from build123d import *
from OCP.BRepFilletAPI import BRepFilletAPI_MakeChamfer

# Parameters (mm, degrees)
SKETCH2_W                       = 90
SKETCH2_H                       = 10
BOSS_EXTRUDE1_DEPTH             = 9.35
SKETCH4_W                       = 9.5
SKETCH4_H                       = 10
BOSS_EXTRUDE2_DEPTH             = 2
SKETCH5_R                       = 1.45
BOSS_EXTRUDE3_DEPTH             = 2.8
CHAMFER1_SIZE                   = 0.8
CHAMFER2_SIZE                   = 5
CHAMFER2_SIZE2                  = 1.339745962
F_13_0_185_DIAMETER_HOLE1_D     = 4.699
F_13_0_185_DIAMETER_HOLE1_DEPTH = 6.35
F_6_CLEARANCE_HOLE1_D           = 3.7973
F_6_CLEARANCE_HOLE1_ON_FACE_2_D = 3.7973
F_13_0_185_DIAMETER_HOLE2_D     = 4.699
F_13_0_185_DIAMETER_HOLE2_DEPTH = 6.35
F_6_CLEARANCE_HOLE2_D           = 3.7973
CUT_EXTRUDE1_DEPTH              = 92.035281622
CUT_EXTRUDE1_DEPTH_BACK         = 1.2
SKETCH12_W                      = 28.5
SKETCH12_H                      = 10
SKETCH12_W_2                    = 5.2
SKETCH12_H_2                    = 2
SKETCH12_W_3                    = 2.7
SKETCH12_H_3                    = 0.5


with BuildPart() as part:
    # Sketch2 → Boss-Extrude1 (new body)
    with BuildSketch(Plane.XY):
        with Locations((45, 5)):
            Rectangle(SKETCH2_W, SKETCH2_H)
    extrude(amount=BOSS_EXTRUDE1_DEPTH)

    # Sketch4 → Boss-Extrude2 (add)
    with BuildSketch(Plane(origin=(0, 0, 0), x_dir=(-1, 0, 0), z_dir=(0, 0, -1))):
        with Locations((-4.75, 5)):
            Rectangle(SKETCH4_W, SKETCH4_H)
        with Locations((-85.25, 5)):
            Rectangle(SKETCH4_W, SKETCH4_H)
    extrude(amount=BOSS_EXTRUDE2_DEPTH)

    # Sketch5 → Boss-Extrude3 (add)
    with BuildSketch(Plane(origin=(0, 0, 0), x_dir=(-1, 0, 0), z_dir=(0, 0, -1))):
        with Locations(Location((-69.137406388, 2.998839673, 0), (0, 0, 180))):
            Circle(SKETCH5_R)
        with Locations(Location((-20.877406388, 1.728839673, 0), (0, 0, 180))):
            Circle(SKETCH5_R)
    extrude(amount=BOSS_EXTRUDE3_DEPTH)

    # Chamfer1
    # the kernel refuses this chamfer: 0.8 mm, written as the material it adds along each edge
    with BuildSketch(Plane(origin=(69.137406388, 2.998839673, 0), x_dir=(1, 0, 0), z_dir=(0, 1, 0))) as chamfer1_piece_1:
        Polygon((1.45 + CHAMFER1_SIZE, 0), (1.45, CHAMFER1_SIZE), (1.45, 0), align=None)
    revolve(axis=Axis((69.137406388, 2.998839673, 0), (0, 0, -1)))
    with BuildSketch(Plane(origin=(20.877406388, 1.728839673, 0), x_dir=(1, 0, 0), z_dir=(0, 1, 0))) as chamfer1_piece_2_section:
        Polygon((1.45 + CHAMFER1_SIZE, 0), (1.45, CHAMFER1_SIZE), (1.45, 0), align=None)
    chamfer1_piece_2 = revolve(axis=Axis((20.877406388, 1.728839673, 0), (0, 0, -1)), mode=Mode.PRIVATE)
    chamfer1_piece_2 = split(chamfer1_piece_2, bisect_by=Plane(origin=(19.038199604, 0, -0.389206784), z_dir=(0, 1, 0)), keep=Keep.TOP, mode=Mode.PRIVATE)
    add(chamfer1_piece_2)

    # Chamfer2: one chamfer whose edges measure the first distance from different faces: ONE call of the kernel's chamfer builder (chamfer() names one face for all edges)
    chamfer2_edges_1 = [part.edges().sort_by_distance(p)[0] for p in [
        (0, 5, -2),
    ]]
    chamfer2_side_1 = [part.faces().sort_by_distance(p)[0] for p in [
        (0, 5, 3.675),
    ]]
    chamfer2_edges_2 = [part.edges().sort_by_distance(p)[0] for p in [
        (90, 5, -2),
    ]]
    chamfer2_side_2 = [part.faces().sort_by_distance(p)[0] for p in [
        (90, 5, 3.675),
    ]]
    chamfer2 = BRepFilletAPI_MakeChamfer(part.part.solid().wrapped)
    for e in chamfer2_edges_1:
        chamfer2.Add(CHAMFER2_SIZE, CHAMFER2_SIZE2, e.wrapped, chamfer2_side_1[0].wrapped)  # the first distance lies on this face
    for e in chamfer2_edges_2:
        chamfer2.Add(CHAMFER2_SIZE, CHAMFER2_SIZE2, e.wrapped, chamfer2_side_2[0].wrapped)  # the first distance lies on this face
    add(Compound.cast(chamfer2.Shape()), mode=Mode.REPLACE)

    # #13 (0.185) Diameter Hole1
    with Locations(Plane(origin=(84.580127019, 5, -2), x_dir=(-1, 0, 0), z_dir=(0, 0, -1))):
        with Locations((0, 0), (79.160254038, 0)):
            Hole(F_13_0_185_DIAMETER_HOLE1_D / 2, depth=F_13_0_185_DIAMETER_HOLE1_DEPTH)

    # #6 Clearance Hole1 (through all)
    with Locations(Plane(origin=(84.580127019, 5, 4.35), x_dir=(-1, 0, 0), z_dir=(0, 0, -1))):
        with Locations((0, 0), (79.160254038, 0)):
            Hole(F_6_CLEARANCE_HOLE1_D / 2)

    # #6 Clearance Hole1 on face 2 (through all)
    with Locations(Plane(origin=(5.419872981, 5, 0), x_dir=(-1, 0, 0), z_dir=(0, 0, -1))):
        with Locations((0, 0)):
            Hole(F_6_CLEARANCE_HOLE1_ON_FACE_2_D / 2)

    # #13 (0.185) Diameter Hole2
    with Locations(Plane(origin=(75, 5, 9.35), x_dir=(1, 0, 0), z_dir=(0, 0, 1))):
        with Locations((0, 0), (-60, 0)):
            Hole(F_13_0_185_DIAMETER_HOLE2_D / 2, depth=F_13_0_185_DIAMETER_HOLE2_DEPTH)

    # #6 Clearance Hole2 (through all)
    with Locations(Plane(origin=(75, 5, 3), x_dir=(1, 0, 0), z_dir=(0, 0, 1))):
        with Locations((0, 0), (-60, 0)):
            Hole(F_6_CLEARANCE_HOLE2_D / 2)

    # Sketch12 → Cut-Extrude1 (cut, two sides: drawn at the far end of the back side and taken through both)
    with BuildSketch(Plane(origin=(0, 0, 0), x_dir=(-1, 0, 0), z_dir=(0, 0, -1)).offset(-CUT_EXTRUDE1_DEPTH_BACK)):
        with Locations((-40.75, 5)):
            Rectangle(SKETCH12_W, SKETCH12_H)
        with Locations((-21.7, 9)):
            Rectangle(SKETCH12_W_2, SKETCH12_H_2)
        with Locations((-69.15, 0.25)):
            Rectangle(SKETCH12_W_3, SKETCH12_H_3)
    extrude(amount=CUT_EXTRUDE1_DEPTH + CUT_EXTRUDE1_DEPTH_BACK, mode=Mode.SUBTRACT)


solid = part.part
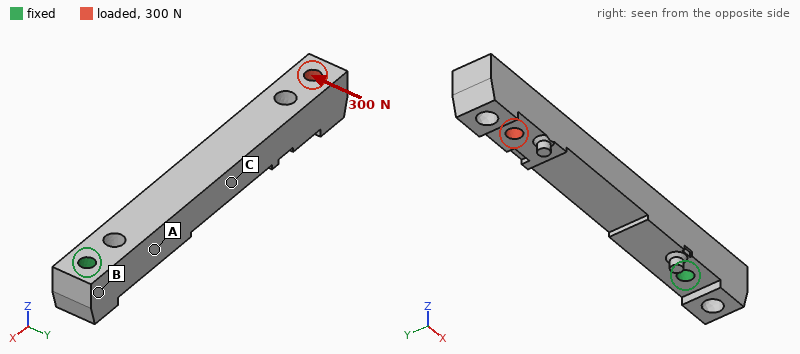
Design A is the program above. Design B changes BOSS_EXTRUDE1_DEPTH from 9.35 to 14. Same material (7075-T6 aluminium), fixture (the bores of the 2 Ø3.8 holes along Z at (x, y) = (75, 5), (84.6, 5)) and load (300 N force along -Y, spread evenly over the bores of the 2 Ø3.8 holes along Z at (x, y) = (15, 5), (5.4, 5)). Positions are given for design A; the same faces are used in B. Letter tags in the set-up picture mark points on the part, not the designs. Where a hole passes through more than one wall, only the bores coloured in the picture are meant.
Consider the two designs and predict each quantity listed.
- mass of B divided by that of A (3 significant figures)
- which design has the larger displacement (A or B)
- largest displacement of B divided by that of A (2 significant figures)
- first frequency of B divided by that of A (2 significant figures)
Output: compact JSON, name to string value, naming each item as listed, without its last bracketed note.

{"mass of B divided by that of A": "1.50", "which design has the larger displacement": "A", "largest displacement of B divided by that of A": "0.72", "first frequency of B divided by that of A": "1.1"}
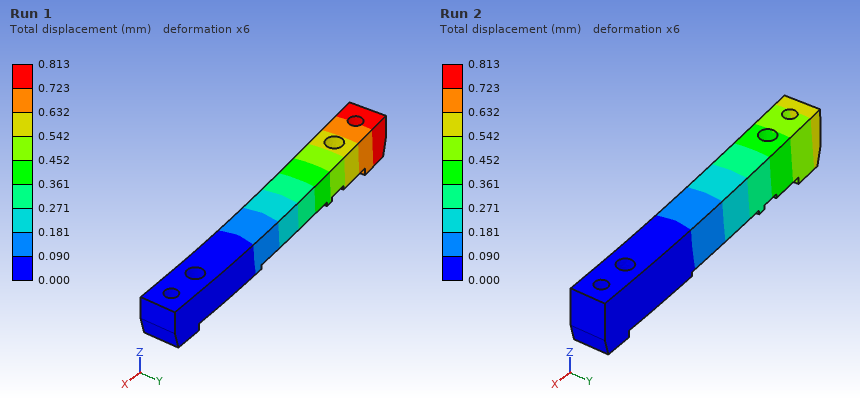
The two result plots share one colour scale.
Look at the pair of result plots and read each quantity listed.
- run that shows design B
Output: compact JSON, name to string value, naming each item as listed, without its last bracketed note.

{"run that shows design B": "Run 2"}
